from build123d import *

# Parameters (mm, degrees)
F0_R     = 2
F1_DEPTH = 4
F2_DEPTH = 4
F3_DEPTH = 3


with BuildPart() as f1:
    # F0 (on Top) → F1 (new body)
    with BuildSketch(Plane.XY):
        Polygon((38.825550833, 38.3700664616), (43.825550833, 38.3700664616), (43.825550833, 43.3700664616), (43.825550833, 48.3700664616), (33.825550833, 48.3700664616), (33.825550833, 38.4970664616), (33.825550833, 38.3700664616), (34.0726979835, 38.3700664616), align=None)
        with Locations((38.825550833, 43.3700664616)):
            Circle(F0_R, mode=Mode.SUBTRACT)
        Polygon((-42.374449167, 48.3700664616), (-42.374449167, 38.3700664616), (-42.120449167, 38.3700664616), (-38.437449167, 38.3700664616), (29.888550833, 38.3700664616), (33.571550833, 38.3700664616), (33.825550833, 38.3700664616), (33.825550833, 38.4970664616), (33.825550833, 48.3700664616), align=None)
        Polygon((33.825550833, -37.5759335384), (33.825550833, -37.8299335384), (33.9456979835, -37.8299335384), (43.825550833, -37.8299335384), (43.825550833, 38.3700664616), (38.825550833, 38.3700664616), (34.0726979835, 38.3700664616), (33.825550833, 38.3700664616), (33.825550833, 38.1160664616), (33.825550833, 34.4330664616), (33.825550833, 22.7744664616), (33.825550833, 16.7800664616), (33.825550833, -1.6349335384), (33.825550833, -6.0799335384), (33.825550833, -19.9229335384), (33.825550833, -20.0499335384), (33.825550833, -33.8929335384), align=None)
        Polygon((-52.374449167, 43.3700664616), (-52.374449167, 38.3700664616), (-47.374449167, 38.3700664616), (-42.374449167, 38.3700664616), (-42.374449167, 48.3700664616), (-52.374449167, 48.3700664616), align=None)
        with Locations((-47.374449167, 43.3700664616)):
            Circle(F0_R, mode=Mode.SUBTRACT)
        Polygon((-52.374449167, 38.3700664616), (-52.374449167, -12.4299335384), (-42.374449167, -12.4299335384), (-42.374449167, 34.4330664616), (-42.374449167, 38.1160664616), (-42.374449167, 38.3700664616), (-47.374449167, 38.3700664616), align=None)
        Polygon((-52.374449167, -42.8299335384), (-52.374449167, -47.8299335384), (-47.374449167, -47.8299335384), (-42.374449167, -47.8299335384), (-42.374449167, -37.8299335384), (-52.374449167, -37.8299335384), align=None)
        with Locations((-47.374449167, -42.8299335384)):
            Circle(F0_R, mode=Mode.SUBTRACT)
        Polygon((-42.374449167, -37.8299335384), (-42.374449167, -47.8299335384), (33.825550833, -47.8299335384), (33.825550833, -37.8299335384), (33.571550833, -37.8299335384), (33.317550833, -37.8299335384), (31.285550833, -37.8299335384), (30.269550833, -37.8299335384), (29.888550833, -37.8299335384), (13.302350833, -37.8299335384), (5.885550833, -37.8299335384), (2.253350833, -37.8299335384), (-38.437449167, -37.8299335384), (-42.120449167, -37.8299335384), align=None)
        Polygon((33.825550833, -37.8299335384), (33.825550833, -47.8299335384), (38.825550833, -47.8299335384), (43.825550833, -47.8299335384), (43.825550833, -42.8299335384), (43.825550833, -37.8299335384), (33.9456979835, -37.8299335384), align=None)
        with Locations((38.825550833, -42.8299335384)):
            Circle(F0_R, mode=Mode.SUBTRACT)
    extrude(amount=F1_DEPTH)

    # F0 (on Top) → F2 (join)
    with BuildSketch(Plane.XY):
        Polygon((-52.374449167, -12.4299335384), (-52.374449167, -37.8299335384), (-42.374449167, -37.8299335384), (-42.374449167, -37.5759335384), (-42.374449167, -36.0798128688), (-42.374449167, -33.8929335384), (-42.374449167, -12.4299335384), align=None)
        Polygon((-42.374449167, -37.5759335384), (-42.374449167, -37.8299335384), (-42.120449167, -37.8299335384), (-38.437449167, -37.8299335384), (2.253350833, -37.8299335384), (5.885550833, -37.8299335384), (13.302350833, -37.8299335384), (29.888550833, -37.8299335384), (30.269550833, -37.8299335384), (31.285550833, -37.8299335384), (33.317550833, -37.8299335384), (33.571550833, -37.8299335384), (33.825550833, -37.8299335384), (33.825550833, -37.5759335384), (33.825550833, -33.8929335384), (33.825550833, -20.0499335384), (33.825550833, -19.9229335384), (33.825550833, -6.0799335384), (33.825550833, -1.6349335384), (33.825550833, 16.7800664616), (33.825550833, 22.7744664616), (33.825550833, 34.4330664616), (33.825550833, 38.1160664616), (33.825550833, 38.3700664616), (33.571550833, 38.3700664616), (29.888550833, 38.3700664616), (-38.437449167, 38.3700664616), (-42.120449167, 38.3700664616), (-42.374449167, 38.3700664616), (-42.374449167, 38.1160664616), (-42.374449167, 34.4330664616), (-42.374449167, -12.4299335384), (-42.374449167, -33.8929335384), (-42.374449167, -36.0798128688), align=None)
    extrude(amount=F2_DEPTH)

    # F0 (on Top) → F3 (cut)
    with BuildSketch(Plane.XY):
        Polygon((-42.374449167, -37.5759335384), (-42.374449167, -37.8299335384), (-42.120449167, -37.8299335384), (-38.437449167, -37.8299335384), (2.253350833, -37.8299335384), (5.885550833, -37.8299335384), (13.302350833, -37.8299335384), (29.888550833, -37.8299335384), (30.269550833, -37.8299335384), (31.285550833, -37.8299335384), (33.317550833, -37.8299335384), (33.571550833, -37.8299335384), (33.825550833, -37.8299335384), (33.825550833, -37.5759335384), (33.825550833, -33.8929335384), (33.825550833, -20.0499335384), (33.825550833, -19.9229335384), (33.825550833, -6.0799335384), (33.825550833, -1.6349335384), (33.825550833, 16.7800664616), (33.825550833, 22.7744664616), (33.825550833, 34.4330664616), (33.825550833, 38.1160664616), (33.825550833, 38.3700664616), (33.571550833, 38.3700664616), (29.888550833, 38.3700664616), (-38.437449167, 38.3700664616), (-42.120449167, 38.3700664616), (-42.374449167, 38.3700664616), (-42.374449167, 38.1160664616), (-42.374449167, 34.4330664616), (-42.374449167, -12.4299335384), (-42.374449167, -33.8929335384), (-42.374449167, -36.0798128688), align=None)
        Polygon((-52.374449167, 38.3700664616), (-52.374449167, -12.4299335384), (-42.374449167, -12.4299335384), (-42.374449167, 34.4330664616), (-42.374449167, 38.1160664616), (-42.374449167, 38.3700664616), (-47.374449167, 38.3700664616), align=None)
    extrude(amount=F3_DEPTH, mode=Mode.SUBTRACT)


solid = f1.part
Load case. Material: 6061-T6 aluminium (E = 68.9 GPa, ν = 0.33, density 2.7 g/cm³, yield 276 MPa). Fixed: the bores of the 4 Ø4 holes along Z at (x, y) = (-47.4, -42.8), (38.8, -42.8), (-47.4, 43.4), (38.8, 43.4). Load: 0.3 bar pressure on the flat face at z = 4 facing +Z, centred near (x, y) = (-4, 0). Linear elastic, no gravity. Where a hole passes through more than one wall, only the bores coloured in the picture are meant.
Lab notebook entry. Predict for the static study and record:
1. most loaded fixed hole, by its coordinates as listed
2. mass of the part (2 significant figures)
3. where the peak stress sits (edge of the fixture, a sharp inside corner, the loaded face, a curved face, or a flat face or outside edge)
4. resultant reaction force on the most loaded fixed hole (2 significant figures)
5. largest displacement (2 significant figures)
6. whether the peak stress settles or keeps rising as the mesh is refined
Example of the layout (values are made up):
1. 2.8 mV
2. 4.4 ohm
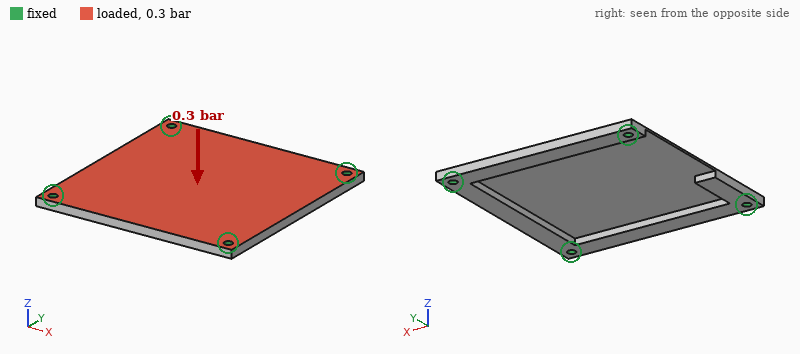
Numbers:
1. (-47.4, -42.8)
2. 48 g
3. edge of the fixture
4. 210 N
5. 0.32 mm
6. keeps rising
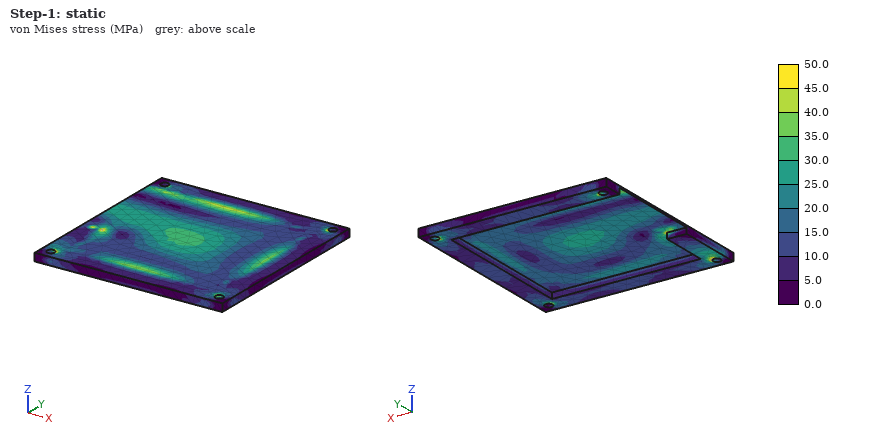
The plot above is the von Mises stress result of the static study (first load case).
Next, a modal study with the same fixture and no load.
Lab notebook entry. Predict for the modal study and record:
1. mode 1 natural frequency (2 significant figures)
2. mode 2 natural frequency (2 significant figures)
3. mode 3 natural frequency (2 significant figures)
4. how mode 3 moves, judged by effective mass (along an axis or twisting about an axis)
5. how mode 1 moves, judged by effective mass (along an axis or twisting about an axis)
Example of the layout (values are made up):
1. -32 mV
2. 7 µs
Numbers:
1. 1200 Hz
2. 1800 Hz
3. 2300 Hz
4. twisting about X
5. along Z
